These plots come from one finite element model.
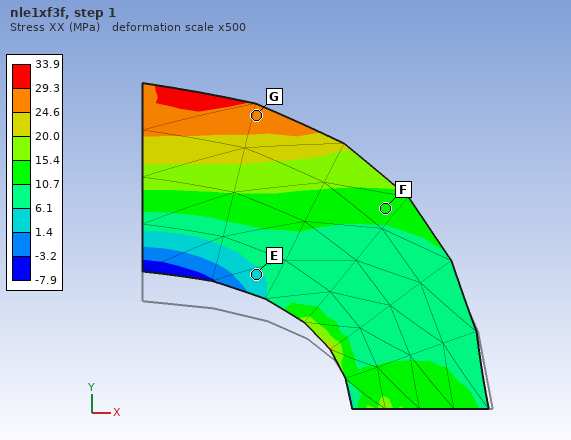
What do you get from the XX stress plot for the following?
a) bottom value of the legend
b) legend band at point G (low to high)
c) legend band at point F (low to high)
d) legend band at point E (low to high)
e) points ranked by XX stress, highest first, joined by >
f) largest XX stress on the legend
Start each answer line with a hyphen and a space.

- -7.9 MPa
- 24.6 to 29.3 MPa
- 10.7 to 15.4 MPa
- 1.4 to 6.1 MPa
- G > F > E
- 33.9 MPa
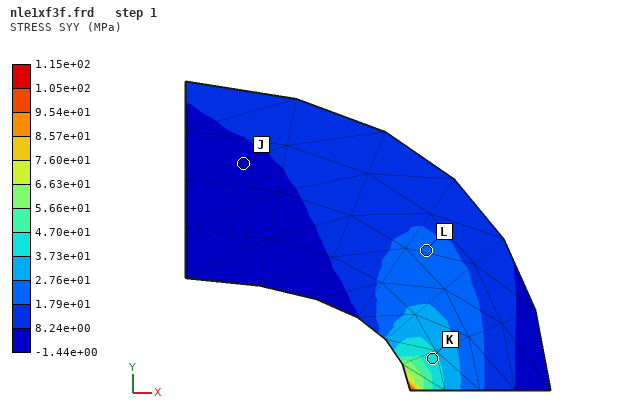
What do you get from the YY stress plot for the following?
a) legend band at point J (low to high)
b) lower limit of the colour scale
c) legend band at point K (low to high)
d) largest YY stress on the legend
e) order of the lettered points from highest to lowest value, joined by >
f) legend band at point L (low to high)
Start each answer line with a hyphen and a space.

- -1.44e+00 to 8.24e+00 MPa
- -1.44e+00 MPa
- 3.73e+01 to 4.70e+01 MPa
- 1.15e+02 MPa
- K > L > J
- 1.79e+01 to 2.76e+01 MPa
